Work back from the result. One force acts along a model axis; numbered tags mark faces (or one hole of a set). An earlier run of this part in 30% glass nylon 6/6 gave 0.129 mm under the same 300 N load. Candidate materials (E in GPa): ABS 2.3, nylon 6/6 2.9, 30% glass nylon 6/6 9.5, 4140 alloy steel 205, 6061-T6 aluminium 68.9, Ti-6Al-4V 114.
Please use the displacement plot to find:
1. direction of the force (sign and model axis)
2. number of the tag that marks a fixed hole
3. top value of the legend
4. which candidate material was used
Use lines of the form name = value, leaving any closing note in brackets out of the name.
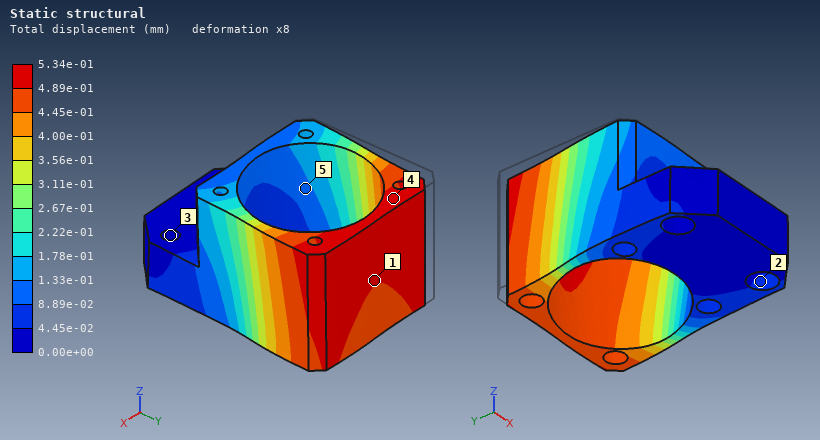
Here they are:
direction of the force = +X
number of the tag that marks a fixed hole = 3
top value of the legend = 5.34e-01 mm
which candidate material was used = ABS
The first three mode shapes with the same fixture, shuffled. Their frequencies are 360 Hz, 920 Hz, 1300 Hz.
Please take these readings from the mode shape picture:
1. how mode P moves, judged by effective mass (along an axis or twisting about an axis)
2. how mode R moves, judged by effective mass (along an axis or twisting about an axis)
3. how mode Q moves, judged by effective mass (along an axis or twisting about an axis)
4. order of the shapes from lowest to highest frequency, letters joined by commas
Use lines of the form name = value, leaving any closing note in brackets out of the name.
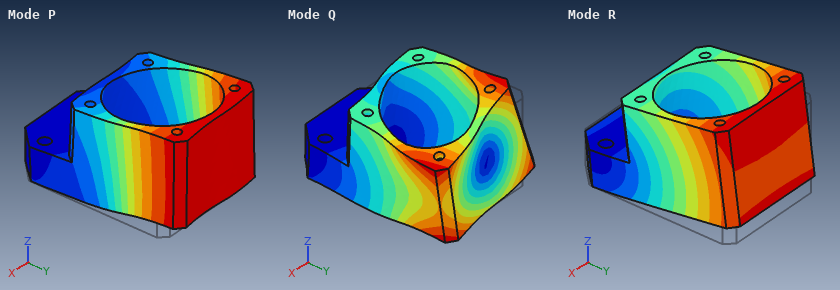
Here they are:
how mode P moves, judged by effective mass = along X
how mode R moves, judged by effective mass = along Z
how mode Q moves, judged by effective mass = twisting about Y
order of the shapes from lowest to highest frequency, letters joined by commas = R, P, Q
